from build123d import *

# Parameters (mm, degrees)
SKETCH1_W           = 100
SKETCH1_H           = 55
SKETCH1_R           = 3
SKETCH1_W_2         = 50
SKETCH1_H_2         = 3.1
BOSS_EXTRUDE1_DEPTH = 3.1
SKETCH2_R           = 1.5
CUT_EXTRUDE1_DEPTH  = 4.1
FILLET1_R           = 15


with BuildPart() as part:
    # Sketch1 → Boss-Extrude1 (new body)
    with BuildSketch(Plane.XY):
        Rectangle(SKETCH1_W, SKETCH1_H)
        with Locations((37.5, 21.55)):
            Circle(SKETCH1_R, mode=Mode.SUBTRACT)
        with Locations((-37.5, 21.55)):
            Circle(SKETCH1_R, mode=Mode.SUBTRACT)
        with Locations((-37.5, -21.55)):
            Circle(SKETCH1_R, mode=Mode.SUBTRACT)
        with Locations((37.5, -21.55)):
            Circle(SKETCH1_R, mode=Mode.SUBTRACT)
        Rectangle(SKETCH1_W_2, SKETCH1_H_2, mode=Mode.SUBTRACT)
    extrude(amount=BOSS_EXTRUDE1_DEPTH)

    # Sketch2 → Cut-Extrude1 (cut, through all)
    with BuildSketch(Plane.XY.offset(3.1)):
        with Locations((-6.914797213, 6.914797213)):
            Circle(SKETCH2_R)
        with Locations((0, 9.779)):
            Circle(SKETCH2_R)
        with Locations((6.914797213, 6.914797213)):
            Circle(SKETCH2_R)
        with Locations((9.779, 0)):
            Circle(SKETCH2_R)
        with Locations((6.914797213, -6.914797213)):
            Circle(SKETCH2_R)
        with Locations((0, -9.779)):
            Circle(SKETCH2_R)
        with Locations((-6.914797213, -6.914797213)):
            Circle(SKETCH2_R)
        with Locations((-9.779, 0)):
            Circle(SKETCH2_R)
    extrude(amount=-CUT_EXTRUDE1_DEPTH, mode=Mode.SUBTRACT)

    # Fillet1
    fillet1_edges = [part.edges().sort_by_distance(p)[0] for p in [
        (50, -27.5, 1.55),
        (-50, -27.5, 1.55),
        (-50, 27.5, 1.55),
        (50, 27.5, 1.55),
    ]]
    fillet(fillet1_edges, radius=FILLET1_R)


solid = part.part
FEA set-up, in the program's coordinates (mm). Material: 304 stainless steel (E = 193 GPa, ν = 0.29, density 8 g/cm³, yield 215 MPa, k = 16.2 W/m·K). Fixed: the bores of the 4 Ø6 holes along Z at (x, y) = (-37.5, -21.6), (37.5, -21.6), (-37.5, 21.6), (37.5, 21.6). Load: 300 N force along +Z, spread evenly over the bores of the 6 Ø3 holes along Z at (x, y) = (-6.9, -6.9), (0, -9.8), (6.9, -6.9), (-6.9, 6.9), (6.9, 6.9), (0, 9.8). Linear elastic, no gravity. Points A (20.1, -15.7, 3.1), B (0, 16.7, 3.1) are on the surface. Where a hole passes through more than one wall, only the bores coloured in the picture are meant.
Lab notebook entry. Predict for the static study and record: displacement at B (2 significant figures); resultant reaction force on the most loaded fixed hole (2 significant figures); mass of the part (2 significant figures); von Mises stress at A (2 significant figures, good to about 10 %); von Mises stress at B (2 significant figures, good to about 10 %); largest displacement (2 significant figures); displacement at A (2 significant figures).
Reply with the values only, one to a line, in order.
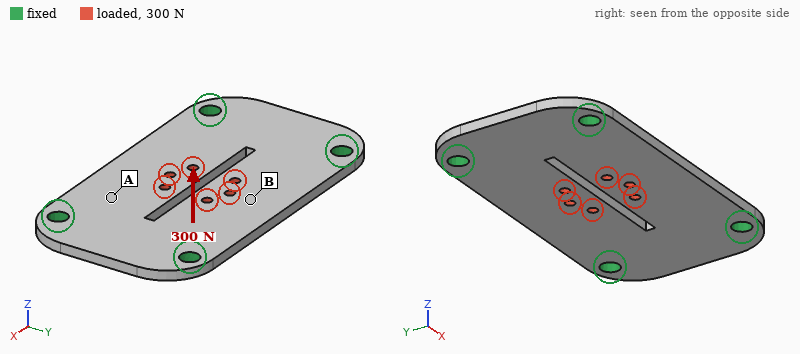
26 µm
75 N
120 g
9.7 MPa
26 MPa
42 µm
13 µm
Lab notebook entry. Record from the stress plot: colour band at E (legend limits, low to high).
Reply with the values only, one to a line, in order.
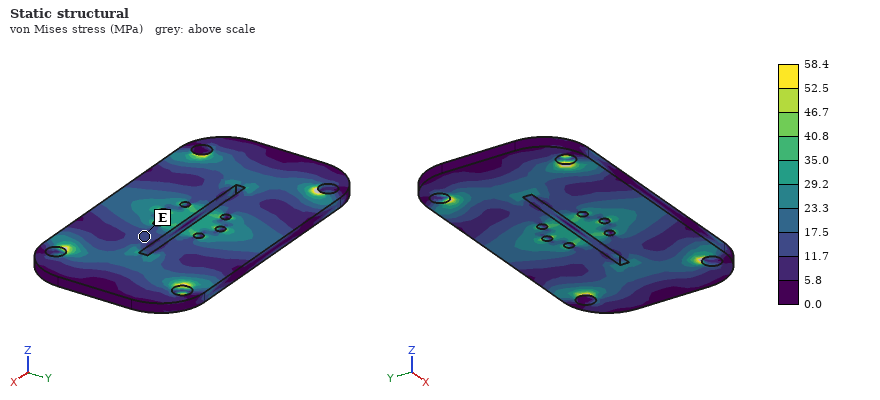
11.7 to 17.5 MPa
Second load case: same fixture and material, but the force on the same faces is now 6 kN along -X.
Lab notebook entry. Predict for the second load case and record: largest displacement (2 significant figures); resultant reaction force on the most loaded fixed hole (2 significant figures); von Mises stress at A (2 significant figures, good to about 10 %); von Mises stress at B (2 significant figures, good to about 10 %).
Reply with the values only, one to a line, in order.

6.1 µm
1.5 kN
24 MPa
18 MPa
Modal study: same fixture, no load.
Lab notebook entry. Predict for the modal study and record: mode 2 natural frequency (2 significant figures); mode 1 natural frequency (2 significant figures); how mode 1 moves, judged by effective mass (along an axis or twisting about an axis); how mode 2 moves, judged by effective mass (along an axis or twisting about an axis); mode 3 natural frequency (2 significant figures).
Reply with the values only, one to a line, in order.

3400 Hz
2700 Hz
along Z
twisting about X
5500 Hz
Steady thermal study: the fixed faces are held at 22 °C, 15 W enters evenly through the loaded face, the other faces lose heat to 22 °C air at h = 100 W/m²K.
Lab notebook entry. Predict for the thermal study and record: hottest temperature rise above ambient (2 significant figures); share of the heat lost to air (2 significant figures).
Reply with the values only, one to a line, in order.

52 K
86 %
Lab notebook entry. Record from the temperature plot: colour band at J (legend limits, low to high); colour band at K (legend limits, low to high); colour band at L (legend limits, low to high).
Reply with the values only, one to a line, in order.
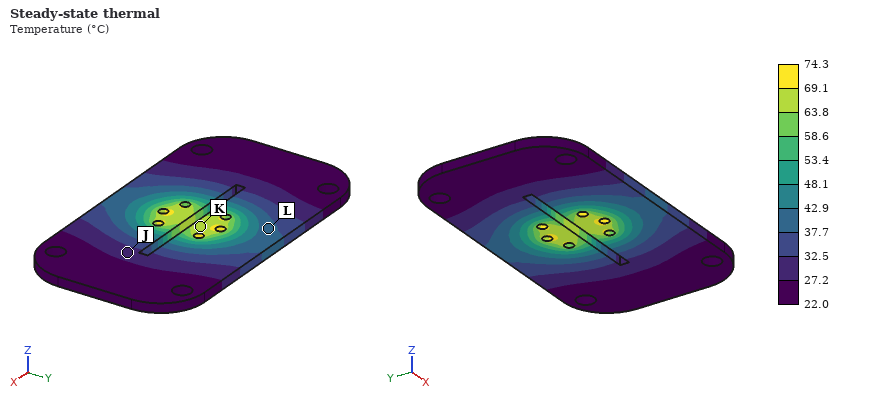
27.2 to 32.5 °C
63.8 to 69.1 °C
37.7 to 42.9 °C
